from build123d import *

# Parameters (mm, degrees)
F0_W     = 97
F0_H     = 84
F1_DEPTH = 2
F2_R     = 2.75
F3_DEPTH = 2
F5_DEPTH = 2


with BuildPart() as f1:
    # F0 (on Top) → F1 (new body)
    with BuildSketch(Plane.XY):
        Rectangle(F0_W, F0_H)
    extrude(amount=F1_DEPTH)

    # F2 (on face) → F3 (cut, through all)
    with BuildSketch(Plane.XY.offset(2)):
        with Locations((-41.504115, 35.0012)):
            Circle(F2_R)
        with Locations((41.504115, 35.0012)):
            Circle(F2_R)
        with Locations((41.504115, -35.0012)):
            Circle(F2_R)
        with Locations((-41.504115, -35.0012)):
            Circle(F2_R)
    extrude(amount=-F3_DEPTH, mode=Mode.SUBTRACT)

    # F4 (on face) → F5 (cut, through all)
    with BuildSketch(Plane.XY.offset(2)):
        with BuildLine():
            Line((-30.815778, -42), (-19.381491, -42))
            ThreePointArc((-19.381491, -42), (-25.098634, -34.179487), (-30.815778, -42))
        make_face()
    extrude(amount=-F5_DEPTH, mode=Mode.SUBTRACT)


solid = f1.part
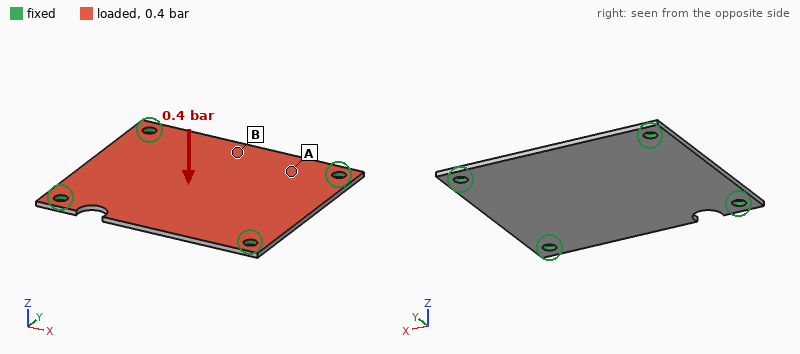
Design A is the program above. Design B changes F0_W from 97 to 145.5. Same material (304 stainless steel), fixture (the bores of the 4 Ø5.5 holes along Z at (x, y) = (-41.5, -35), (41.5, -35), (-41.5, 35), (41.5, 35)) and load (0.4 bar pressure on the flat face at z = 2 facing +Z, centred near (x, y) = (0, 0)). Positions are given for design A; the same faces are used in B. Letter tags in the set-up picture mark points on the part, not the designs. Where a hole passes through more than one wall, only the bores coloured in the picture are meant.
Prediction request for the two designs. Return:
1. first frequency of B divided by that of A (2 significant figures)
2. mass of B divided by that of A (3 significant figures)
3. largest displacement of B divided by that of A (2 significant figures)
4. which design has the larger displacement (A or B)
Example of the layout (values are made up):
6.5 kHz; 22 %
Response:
0.97; 1.51; 0.83; A
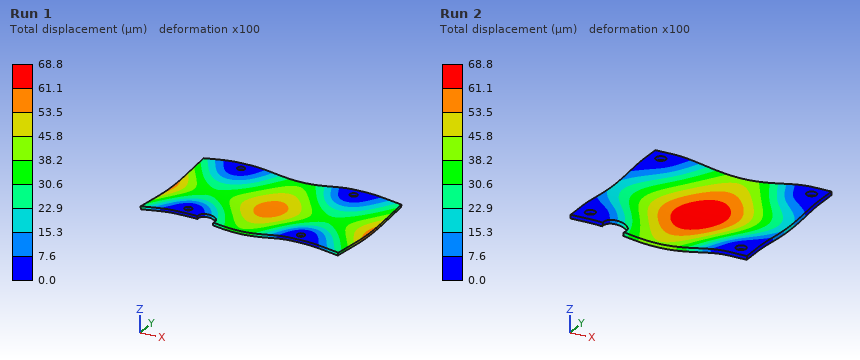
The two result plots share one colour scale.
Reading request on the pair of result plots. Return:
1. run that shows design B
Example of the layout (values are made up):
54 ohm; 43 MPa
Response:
Run 1
